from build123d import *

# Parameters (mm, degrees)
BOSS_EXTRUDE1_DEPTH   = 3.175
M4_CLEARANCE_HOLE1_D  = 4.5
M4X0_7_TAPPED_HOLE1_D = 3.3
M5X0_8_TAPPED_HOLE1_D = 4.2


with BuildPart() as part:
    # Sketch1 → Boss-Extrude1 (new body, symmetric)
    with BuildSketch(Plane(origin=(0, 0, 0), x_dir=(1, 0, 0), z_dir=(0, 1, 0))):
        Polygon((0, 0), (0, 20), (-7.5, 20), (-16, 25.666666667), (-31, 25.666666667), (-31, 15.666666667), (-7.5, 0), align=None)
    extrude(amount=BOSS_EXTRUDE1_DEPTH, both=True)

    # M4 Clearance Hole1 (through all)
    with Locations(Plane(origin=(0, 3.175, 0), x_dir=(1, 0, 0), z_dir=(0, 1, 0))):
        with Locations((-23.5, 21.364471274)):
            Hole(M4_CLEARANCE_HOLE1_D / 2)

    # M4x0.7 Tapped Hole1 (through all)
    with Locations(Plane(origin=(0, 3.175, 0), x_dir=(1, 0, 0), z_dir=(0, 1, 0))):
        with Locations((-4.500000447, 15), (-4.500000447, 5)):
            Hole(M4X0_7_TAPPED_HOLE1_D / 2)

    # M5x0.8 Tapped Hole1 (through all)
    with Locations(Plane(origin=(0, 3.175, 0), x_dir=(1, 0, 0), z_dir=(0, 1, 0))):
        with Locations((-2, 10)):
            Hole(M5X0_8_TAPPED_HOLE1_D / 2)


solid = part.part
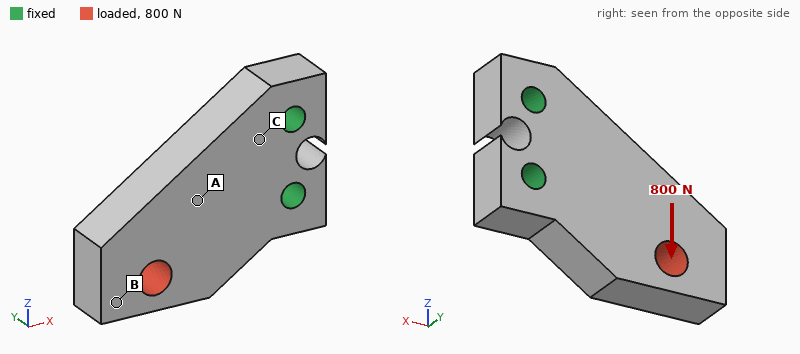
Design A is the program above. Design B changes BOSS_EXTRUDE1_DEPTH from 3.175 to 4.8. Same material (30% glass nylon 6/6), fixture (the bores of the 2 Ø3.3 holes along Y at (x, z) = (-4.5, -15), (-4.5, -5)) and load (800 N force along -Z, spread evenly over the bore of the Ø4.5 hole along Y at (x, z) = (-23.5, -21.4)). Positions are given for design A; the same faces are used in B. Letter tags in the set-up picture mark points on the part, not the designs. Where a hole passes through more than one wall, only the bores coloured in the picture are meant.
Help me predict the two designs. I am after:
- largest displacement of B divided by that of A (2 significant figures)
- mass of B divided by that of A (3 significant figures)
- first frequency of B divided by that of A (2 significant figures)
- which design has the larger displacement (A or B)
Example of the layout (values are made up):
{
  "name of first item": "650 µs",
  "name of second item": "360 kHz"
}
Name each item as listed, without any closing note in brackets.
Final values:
{
  "largest displacement of B divided by that of A": "0.66",
  "mass of B divided by that of A": "1.51",
  "first frequency of B divided by that of A": "1.4",
  "which design has the larger displacement": "A"
}
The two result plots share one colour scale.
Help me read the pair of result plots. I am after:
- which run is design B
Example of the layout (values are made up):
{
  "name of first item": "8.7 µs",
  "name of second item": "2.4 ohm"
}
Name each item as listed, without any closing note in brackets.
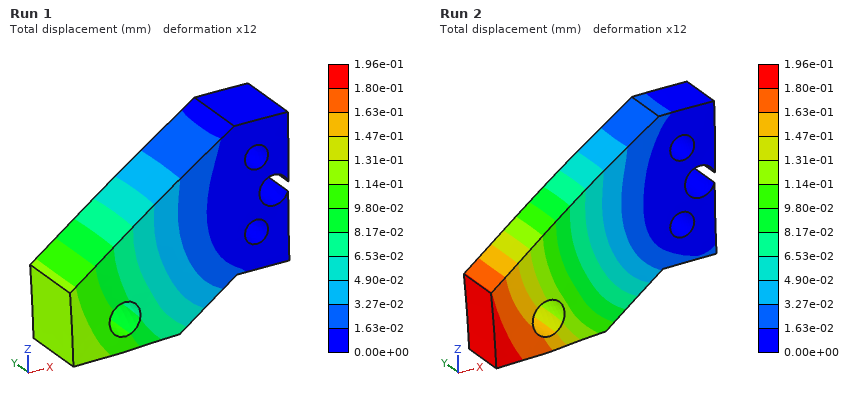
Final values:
{
  "which run is design B": "Run 1"
}
